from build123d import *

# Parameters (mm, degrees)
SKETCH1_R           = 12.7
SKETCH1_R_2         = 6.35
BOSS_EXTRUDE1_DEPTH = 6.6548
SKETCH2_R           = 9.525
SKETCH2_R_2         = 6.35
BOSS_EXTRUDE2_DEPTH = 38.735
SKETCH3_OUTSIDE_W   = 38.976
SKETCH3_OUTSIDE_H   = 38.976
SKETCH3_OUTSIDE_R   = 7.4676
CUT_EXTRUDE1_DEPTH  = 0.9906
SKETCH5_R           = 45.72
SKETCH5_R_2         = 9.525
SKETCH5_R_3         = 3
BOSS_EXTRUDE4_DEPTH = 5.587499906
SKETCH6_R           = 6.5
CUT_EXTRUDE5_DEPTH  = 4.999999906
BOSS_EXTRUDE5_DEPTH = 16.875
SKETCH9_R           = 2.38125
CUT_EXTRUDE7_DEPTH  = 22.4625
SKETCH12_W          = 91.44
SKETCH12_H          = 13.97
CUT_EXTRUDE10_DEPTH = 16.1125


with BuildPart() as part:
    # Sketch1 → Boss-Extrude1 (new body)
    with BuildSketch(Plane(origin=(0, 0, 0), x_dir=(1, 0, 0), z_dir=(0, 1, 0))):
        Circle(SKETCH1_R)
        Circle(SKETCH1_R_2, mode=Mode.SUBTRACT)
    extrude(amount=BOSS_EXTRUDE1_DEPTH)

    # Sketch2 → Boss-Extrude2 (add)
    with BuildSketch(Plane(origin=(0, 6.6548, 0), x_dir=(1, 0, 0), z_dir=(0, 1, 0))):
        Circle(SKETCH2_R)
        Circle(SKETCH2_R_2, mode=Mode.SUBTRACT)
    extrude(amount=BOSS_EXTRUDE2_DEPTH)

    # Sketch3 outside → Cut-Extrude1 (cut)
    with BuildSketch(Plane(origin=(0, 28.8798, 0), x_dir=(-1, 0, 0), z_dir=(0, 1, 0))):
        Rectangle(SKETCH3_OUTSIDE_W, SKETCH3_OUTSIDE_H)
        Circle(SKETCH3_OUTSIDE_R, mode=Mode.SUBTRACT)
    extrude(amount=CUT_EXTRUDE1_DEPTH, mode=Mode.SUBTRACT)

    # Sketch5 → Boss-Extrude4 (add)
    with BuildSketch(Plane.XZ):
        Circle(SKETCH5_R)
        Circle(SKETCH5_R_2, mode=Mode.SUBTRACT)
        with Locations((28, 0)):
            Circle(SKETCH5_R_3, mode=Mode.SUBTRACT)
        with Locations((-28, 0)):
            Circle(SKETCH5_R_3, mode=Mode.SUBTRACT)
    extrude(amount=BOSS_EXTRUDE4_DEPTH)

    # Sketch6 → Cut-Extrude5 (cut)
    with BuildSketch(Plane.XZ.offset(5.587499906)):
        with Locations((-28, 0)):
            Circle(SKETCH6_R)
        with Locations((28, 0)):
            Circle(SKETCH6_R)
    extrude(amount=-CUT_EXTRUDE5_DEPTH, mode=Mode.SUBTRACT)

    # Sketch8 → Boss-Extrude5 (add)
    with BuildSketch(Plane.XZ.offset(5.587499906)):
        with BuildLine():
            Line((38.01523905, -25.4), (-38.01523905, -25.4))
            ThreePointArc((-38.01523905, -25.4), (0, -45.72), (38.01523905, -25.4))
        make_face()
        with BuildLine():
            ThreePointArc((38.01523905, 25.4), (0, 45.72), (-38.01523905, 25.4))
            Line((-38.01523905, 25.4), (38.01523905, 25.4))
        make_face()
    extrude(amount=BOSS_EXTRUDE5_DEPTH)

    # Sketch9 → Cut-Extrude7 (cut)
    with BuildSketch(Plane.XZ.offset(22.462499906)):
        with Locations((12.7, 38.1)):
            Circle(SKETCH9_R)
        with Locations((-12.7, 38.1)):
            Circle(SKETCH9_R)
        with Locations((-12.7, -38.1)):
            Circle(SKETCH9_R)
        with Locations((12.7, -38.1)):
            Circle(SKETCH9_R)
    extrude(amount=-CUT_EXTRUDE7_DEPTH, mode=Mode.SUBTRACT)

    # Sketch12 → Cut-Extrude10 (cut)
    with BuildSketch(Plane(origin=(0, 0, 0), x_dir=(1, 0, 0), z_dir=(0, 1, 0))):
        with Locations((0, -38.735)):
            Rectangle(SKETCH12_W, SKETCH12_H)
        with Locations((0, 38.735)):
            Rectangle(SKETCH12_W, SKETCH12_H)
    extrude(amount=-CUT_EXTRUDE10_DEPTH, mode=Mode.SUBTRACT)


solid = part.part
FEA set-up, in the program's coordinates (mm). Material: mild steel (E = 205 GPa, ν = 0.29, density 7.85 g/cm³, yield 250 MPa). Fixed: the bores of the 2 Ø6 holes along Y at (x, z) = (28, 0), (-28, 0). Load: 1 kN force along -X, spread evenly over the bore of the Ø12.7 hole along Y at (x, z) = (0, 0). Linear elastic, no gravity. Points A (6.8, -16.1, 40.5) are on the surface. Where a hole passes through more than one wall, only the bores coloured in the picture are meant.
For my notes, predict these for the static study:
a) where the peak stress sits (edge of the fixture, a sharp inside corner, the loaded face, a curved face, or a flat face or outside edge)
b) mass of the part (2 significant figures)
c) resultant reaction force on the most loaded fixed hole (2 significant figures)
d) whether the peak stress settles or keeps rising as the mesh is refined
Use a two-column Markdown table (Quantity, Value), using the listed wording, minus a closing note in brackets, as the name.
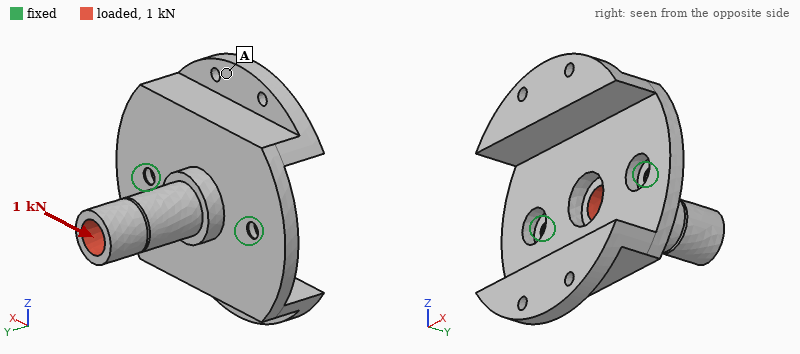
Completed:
| Quantity | Value |
|---|---|
| where the peak stress sits | edge of the fixture |
| mass of the part | 460 g |
| resultant reaction force on the most loaded fixed hole | 650 N |
| whether the peak stress settles or keeps rising as the mesh is refined | keeps rising |
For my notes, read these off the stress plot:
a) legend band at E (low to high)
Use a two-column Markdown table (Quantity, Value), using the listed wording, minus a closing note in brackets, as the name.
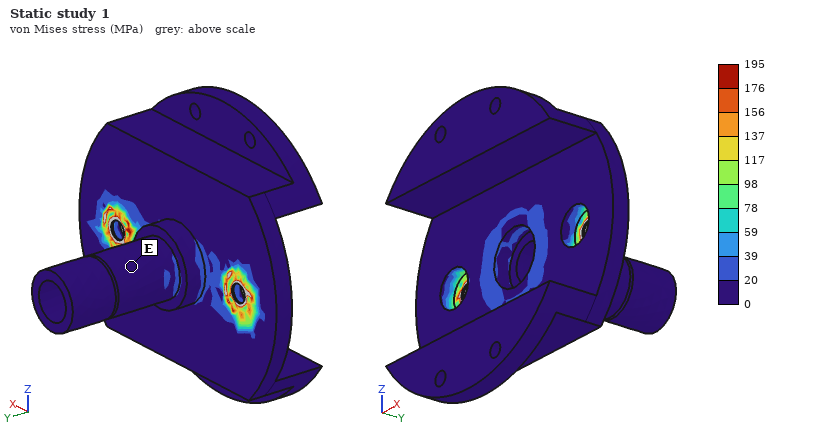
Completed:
| Quantity | Value |
|---|---|
| legend band at E | 0 to 20 MPa |
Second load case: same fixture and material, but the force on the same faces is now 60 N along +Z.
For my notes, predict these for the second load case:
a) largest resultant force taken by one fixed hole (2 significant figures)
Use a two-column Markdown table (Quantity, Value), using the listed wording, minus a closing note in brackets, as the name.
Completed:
| Quantity | Value |
|---|---|
| largest resultant force taken by one fixed hole | 30 N |
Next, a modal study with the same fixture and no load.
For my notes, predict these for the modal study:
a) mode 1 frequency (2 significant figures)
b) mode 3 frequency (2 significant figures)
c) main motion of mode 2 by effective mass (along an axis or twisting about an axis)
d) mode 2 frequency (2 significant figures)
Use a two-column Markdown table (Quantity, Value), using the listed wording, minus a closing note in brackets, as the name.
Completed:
| Quantity | Value |
|---|---|
| mode 1 frequency | 240 Hz |
| mode 3 frequency | 2000 Hz |
| main motion of mode 2 by effective mass | along Y |
| mode 2 frequency | 1500 Hz |
